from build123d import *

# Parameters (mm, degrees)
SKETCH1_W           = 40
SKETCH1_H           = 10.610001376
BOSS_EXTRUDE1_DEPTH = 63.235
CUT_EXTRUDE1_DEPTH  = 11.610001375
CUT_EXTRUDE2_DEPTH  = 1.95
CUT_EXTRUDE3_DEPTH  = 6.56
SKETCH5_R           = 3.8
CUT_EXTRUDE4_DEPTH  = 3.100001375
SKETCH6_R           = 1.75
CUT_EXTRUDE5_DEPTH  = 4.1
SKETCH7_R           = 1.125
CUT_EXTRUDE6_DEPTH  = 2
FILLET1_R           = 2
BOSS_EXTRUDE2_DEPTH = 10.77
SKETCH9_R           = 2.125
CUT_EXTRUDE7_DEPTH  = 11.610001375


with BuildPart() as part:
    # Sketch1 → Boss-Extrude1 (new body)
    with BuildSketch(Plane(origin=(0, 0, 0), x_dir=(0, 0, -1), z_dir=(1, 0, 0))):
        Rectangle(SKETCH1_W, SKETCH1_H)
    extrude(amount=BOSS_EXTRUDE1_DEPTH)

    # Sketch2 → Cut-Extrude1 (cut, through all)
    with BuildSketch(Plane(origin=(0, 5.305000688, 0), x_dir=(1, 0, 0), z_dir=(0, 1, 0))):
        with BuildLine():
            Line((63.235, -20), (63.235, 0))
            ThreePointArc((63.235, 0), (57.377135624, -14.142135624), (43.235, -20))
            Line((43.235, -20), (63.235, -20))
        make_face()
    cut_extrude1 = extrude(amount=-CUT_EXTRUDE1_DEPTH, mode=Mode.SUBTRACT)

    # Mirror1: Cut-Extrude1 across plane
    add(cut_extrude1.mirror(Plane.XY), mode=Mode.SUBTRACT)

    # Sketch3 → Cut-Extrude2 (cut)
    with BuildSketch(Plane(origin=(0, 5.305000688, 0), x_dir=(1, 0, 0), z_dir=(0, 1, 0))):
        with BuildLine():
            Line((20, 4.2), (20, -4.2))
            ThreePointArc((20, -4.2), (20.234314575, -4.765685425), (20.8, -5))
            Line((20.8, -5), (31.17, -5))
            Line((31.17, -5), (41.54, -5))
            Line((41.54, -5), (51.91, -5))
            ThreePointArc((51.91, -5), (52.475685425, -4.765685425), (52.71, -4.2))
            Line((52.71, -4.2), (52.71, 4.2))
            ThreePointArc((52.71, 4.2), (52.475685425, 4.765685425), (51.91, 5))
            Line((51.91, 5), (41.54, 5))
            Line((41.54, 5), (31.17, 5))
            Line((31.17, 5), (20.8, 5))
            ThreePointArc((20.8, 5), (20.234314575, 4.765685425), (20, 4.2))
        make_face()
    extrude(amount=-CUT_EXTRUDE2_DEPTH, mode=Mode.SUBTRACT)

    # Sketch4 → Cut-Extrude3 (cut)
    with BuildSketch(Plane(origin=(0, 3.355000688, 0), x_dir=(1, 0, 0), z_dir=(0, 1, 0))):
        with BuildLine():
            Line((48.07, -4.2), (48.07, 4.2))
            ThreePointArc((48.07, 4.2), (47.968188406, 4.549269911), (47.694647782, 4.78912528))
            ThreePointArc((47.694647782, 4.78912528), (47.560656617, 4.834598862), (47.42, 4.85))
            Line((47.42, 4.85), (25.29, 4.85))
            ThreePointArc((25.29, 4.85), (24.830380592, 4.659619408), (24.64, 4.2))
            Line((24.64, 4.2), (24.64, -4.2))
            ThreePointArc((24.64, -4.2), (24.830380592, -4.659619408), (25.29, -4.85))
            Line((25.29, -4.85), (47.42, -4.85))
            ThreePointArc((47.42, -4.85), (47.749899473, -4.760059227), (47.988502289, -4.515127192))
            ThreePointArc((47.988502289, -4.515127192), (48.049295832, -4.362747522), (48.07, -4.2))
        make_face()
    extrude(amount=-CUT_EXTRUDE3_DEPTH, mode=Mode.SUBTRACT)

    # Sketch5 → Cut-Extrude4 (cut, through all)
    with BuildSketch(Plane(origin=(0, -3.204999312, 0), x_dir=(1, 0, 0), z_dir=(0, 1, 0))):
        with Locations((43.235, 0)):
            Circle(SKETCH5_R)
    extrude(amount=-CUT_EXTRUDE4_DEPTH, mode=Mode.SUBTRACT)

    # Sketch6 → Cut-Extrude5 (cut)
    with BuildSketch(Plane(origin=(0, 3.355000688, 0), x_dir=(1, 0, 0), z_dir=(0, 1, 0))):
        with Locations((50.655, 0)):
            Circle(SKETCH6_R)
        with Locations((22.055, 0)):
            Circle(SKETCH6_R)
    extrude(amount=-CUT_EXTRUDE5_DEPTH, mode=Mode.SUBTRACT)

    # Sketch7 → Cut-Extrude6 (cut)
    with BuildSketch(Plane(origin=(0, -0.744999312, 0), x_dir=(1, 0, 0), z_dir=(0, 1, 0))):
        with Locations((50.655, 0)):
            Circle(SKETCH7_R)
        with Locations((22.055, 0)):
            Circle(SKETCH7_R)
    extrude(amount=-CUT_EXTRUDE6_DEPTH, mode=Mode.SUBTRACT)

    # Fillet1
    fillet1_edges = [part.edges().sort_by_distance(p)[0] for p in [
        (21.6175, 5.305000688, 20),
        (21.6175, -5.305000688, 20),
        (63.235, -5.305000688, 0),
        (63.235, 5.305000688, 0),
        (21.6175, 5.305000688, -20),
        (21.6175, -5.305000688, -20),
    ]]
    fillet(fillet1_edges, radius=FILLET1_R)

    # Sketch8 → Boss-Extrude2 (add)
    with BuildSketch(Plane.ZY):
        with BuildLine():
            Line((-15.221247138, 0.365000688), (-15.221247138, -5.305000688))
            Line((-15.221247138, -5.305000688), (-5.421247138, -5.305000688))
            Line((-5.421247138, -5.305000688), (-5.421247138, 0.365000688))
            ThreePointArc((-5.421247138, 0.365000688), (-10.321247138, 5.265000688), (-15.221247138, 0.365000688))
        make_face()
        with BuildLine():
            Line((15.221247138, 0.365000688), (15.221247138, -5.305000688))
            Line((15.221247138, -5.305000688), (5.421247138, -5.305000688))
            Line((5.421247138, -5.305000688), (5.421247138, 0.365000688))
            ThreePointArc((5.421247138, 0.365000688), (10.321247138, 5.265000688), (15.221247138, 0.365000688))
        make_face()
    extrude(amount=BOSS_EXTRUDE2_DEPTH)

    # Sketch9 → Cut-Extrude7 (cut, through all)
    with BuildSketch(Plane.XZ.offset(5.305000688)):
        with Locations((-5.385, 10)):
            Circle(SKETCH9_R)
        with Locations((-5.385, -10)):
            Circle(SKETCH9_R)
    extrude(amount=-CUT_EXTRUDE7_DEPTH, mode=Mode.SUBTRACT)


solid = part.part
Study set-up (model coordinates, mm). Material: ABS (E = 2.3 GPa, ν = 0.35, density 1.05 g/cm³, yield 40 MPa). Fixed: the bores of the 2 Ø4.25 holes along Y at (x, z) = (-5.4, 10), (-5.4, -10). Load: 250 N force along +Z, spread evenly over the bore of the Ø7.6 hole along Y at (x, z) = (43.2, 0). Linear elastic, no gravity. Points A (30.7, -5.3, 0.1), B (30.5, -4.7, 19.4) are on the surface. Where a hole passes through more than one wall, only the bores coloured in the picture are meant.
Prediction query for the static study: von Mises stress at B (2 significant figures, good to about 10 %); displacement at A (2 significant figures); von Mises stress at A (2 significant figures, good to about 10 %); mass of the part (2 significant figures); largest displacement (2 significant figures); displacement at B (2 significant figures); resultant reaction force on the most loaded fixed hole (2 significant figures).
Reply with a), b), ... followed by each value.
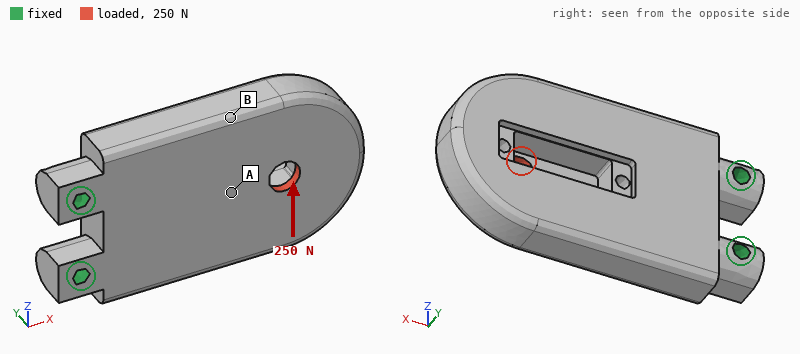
a) 1.7 MPa
b) 0.16 mm
c) 4.8 MPa
d) 25 g
e) 0.31 mm
f) 0.19 mm
g) 520 N
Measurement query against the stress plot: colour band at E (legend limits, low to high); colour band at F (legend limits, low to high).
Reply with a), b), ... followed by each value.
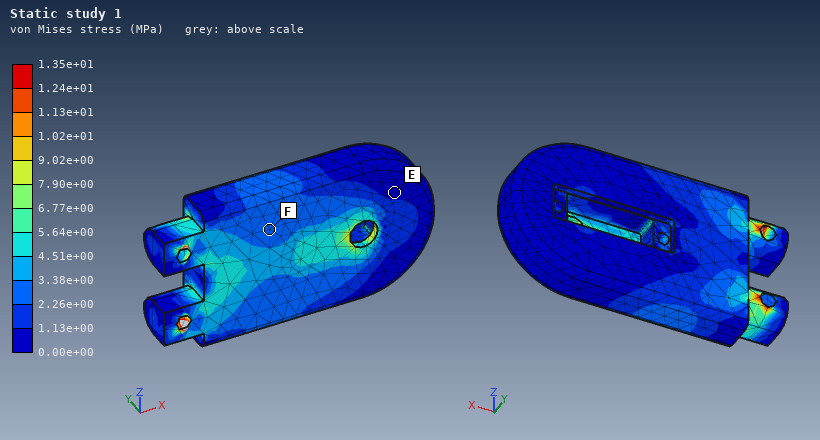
a) 0.00e+00 to 1.13e+00 MPa
b) 2.26e+00 to 3.38e+00 MPa
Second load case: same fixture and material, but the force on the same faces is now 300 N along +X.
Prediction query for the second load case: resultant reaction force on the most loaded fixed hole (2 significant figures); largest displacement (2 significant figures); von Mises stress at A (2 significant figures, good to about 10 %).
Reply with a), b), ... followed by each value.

a) 150 N
b) 0.40 mm
c) 4.3 MPa
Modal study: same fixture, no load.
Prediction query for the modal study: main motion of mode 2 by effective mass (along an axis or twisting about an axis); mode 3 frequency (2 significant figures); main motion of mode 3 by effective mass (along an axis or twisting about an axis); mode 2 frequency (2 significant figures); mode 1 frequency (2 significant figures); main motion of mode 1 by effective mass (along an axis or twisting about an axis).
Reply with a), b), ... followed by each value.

a) along Z
b) 1700 Hz
c) twisting about X
d) 1400 Hz
e) 510 Hz
f) along Y
